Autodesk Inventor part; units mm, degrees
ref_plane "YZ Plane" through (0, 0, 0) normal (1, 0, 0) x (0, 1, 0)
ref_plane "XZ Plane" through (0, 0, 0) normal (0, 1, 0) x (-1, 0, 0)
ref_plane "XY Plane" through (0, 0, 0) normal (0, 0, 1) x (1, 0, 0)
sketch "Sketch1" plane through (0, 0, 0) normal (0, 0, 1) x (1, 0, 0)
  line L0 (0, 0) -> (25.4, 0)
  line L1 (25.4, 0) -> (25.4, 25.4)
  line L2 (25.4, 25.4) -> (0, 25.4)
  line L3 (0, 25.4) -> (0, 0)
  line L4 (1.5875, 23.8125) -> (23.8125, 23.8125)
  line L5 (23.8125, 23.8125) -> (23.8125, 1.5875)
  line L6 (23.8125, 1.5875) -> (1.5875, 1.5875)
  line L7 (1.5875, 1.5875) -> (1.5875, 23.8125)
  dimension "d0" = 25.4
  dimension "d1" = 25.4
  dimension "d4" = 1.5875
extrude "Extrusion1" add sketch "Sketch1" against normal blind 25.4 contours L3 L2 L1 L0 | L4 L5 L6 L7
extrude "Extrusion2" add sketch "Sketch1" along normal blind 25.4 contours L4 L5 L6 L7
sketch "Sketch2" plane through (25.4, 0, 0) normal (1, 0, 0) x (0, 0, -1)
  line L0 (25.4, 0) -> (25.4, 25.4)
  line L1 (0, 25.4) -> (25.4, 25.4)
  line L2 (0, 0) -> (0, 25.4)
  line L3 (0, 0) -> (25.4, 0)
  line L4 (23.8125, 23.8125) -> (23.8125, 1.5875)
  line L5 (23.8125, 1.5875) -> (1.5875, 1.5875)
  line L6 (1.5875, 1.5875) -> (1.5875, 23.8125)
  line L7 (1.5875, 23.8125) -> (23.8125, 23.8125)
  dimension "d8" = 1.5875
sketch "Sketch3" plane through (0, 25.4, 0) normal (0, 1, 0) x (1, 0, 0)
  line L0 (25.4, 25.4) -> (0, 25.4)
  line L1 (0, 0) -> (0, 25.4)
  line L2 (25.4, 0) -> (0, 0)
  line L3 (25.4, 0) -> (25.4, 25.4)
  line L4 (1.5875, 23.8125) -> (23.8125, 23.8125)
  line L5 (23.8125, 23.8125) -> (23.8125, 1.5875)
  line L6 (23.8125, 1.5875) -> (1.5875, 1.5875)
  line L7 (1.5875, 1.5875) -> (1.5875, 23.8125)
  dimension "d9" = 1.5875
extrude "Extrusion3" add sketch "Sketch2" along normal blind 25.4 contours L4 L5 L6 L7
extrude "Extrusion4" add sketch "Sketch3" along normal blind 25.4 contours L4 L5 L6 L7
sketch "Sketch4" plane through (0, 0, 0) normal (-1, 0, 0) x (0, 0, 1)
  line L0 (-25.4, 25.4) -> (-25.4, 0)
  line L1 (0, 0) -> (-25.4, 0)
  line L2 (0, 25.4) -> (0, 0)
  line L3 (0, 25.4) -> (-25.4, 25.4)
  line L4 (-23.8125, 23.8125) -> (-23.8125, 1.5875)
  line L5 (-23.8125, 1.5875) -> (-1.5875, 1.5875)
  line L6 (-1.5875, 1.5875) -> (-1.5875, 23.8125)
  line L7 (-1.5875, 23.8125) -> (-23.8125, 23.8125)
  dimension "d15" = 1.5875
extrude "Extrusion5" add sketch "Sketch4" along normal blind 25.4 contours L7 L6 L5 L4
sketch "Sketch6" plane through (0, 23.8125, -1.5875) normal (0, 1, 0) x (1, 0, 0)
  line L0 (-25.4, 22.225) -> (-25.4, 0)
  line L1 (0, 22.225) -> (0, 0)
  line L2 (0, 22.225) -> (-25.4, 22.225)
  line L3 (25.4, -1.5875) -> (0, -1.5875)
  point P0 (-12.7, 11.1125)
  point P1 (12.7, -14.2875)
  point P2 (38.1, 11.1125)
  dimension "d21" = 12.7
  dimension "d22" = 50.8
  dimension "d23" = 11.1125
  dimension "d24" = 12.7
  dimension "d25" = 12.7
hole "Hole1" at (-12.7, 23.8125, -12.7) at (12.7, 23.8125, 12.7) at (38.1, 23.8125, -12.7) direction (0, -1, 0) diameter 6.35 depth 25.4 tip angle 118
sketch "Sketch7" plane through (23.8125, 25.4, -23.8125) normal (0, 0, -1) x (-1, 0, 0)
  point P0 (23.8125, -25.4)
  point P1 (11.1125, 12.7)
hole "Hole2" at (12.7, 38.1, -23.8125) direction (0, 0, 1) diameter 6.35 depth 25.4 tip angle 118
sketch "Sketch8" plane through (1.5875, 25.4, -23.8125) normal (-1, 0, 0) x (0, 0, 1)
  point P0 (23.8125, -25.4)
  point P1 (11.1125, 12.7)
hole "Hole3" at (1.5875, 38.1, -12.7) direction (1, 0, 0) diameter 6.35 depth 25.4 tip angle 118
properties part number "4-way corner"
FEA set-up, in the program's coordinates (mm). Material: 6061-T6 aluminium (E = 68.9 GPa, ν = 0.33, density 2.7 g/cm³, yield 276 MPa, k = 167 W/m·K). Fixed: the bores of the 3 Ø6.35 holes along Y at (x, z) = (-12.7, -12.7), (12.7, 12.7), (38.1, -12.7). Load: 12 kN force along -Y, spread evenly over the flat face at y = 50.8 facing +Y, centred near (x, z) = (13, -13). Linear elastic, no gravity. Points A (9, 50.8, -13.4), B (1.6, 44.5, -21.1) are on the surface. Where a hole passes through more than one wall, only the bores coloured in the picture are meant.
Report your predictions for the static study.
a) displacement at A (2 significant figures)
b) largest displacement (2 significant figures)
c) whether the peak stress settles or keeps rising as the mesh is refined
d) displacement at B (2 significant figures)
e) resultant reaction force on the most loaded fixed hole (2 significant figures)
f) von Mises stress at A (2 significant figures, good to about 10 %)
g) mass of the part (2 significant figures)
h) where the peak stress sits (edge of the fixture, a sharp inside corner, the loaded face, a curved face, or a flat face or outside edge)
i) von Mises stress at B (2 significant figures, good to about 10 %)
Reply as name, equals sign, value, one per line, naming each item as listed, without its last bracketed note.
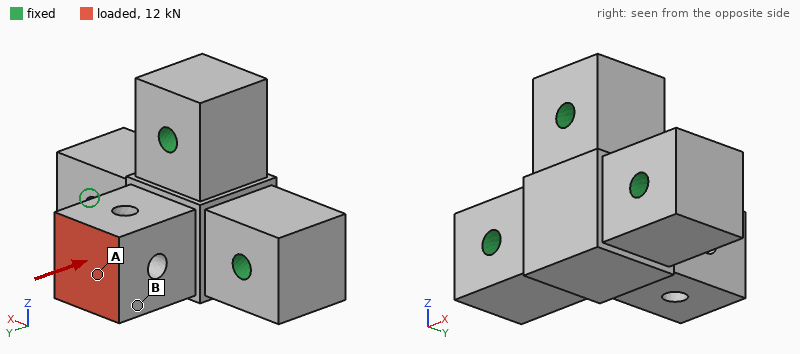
displacement at A = 27 µm
largest displacement = 29 µm
whether the peak stress settles or keeps rising as the mesh is refined = keeps rising
displacement at B = 24 µm
resultant reaction force on the most loaded fixed hole = 4.8 kN
von Mises stress at A = 14 MPa
mass of the part = 170 g
where the peak stress sits = a sharp inside corner
von Mises stress at B = 30 MPa
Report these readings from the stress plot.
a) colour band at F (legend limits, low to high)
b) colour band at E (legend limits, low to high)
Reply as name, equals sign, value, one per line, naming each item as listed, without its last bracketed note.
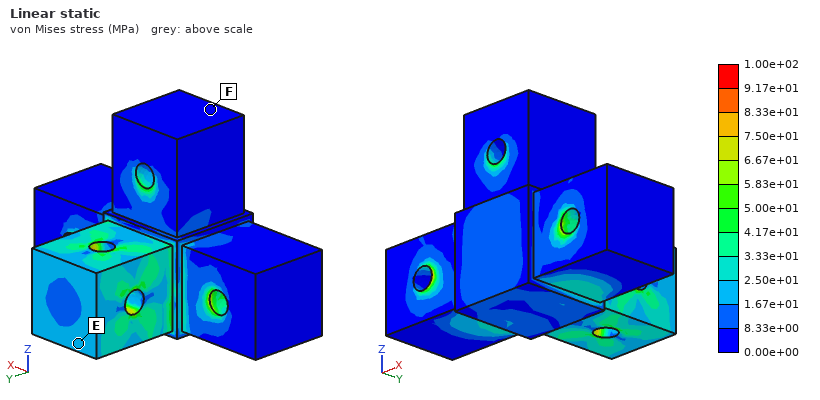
colour band at F = 0.00e+00 to 8.33e+00 MPa
colour band at E = 1.67e+01 to 2.50e+01 MPa
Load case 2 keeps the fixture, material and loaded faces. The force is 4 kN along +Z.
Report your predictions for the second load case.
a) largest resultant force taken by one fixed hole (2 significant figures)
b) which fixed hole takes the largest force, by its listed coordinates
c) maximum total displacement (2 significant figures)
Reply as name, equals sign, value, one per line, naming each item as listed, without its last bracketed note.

largest resultant force taken by one fixed hole = 4.9 kN
which fixed hole takes the largest force, by its listed coordinates = (12.7, 12.7)
maximum total displacement = 71 µm
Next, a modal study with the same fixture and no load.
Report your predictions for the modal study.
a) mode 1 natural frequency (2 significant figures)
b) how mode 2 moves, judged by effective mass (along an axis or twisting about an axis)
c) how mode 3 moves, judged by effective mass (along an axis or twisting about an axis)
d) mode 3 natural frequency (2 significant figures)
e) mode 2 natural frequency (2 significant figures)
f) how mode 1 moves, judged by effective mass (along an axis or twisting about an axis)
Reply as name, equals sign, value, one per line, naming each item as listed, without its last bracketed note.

mode 1 natural frequency = 11 kHz
how mode 2 moves, judged by effective mass = along X
how mode 3 moves, judged by effective mass = along Y
mode 3 natural frequency = 21 kHz
mode 2 natural frequency = 13 kHz
how mode 1 moves, judged by effective mass = along Z
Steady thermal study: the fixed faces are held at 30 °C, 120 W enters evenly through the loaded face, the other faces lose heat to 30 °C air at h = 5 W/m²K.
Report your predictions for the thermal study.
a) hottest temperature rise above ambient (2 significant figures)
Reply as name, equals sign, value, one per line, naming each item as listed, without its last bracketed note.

hottest temperature rise above ambient = 64 K
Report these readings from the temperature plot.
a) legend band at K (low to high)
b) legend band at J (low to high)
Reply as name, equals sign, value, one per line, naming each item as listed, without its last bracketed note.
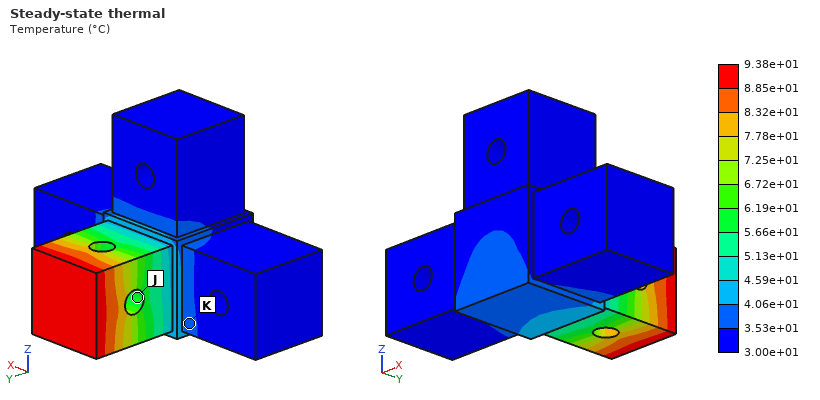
legend band at K = 3.53e+01 to 4.06e+01 °C
legend band at J = 5.66e+01 to 6.19e+01 °C
